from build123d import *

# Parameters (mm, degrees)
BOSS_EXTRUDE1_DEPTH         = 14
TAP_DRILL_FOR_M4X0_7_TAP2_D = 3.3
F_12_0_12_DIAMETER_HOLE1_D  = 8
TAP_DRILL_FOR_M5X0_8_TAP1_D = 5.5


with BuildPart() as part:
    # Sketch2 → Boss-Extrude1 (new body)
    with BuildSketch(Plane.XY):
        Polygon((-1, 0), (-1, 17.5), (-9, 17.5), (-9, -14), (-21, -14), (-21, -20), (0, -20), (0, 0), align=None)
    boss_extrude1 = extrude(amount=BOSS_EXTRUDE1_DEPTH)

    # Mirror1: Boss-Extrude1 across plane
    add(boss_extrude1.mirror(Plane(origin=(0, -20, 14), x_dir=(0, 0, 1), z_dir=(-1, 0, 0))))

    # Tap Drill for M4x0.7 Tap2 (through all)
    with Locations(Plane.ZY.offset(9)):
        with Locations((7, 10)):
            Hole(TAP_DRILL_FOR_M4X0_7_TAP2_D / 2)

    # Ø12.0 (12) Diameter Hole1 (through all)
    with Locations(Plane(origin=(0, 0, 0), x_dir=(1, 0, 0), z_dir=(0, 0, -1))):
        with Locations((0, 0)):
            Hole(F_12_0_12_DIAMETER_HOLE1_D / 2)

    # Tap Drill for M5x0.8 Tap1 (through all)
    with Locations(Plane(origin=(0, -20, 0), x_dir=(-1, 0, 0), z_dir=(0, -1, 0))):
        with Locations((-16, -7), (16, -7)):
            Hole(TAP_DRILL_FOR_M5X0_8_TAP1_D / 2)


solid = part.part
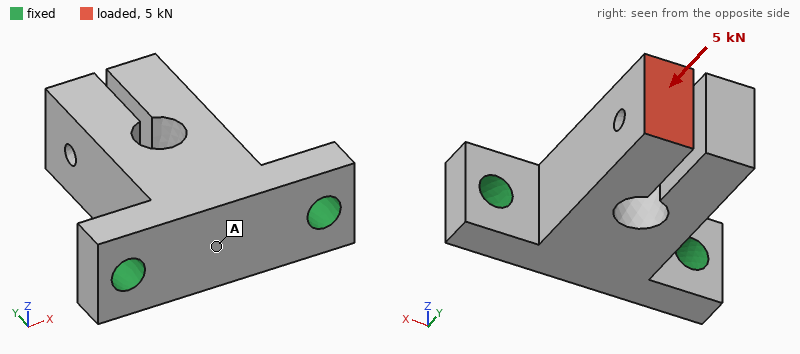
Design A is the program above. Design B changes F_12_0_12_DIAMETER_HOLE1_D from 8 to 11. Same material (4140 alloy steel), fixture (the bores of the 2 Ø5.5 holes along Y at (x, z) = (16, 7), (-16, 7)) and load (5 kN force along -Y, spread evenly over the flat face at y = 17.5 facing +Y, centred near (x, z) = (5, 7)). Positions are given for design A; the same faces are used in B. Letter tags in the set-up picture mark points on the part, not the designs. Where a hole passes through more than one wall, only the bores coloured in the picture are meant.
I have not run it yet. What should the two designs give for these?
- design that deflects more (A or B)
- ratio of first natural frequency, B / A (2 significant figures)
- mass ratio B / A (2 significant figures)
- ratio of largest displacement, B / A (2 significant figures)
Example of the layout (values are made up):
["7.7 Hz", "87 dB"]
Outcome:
["B", "0.98", "0.94", "4.7"]
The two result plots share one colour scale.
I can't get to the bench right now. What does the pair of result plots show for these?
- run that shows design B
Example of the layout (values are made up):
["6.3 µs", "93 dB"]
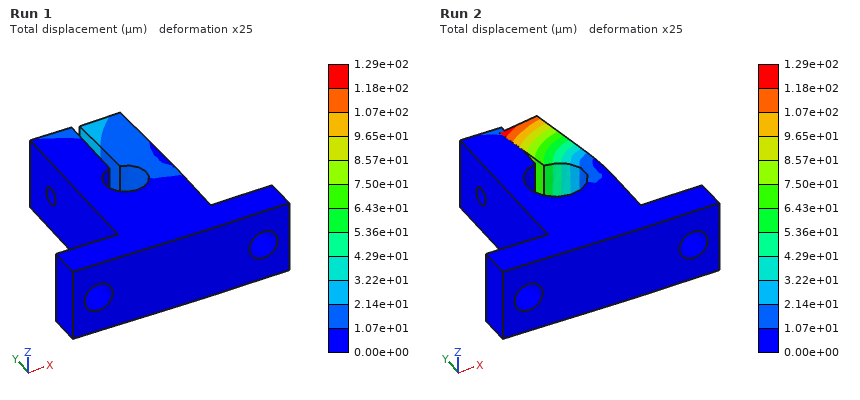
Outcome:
["Run 2"]
